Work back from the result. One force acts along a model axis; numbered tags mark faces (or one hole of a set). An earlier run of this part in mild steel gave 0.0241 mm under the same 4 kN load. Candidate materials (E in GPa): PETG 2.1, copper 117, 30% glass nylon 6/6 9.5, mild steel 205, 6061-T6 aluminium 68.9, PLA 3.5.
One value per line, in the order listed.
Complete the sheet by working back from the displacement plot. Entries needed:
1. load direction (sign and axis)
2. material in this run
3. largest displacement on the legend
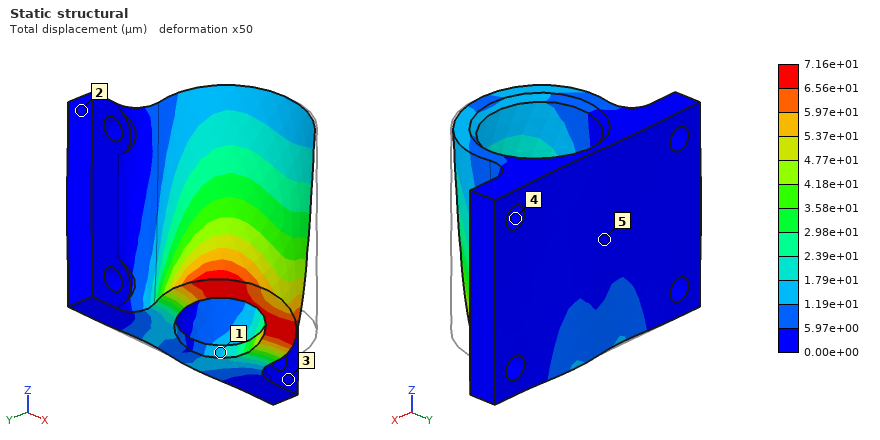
-X
6061-T6 aluminium
7.16e+01 µm
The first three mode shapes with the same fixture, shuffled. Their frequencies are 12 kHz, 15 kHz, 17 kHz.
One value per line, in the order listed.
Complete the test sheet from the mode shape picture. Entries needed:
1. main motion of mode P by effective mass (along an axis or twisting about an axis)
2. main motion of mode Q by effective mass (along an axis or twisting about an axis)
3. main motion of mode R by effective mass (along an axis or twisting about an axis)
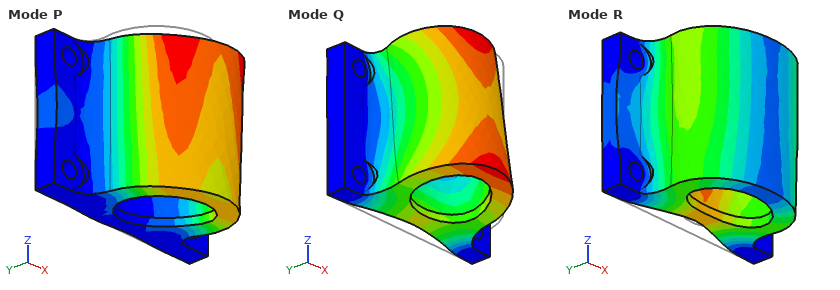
along X
along Z
along Y
